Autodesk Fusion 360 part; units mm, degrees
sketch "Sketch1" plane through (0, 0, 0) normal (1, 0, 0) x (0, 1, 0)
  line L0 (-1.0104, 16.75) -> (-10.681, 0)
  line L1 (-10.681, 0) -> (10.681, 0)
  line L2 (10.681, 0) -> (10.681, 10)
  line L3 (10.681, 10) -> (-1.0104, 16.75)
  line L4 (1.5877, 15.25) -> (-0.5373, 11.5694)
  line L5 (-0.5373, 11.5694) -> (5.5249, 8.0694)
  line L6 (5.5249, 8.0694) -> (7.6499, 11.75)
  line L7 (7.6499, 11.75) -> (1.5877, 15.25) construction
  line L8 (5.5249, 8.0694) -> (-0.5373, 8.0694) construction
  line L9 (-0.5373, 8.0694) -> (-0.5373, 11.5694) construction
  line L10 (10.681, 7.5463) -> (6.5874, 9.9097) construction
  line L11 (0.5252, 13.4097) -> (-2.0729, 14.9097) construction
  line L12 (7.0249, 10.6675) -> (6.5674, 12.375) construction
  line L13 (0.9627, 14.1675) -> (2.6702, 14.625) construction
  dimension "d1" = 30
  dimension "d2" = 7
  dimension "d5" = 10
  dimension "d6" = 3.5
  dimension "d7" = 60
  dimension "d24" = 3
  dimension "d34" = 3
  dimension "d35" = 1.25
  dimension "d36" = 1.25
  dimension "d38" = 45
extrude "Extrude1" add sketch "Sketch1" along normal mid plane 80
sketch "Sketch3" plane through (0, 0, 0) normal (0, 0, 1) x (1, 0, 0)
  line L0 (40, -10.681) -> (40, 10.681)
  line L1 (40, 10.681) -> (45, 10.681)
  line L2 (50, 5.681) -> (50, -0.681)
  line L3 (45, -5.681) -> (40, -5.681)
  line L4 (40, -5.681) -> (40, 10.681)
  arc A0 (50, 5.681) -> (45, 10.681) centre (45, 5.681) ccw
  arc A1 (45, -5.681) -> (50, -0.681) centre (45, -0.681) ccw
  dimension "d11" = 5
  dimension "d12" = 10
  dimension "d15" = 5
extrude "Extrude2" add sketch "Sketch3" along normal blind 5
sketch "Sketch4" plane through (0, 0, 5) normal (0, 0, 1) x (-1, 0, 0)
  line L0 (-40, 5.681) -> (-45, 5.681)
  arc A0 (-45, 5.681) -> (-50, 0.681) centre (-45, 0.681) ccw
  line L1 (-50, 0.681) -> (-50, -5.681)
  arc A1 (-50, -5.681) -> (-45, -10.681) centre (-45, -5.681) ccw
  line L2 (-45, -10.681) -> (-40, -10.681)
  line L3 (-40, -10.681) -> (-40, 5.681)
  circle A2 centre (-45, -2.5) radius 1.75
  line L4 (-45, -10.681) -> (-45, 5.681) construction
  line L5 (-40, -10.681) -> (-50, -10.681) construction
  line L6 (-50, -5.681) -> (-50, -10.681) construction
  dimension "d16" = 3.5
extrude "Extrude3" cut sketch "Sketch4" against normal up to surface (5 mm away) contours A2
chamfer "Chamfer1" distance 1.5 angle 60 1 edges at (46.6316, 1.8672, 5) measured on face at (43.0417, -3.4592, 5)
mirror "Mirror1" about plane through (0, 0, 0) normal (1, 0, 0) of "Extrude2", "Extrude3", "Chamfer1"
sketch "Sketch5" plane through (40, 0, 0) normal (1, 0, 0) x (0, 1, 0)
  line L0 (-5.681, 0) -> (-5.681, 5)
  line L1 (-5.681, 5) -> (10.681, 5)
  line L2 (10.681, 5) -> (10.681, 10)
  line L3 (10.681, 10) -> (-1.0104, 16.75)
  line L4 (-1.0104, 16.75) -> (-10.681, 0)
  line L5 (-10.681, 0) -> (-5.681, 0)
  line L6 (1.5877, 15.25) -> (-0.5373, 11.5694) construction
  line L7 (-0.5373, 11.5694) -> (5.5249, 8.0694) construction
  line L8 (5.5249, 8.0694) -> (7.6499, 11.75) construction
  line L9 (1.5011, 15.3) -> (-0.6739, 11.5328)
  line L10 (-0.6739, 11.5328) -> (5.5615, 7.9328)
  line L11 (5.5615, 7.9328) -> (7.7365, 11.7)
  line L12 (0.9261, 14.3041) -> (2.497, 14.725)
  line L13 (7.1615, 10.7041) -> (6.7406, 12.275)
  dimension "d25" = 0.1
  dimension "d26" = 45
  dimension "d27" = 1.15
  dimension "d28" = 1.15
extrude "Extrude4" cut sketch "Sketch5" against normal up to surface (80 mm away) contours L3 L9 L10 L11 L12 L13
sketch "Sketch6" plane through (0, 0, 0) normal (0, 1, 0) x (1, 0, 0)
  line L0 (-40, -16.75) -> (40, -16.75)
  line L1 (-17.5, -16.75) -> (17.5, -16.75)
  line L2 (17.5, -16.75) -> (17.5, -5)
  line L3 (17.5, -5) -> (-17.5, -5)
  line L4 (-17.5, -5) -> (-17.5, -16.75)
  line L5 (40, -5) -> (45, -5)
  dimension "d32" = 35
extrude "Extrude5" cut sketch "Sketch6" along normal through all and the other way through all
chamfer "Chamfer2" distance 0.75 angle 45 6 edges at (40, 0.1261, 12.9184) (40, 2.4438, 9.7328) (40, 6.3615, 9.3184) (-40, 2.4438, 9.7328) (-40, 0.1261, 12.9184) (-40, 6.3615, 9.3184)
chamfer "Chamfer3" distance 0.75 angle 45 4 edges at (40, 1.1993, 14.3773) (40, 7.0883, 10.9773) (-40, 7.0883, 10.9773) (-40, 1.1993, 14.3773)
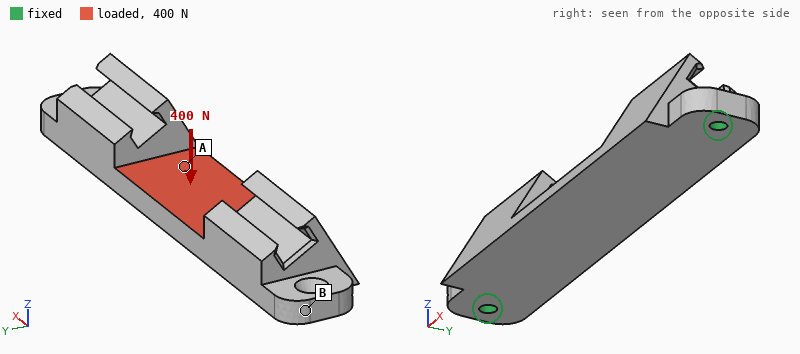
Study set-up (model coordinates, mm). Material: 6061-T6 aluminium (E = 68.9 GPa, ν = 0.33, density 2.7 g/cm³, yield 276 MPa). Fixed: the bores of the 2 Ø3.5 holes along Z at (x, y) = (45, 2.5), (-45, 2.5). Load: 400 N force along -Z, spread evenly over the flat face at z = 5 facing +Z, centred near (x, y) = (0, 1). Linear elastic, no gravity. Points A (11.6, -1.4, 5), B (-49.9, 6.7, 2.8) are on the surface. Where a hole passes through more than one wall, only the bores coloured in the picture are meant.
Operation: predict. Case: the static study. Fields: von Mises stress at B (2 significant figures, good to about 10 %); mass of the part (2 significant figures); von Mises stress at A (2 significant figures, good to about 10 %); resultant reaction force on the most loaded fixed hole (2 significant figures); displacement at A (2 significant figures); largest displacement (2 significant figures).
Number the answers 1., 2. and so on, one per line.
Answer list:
1. 18 MPa
2. 38 g
3. 36 MPa
4. 370 N
5. 0.12 mm
6. 0.14 mm
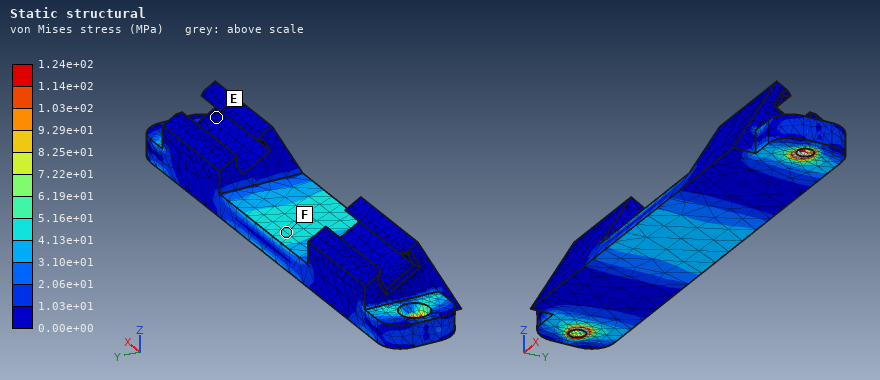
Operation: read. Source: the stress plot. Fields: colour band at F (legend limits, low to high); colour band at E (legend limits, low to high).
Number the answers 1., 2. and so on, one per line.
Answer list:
1. 4.13e+01 to 5.16e+01 MPa
2. 0.00e+00 to 1.03e+01 MPa
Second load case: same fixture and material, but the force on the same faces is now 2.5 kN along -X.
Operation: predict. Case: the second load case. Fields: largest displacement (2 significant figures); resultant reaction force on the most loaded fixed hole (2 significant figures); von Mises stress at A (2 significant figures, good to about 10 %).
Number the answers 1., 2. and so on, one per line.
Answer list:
1. 10 µm
2. 1.3 kN
3. 20 MPa
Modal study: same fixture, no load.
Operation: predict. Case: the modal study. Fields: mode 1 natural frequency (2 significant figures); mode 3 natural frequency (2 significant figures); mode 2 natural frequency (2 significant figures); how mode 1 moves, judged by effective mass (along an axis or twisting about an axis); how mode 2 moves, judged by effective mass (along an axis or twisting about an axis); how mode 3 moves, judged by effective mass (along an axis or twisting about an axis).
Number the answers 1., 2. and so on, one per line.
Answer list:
1. 2300 Hz
2. 6500 Hz
3. 4900 Hz
4. along Z
5. along Y
6. along Y
